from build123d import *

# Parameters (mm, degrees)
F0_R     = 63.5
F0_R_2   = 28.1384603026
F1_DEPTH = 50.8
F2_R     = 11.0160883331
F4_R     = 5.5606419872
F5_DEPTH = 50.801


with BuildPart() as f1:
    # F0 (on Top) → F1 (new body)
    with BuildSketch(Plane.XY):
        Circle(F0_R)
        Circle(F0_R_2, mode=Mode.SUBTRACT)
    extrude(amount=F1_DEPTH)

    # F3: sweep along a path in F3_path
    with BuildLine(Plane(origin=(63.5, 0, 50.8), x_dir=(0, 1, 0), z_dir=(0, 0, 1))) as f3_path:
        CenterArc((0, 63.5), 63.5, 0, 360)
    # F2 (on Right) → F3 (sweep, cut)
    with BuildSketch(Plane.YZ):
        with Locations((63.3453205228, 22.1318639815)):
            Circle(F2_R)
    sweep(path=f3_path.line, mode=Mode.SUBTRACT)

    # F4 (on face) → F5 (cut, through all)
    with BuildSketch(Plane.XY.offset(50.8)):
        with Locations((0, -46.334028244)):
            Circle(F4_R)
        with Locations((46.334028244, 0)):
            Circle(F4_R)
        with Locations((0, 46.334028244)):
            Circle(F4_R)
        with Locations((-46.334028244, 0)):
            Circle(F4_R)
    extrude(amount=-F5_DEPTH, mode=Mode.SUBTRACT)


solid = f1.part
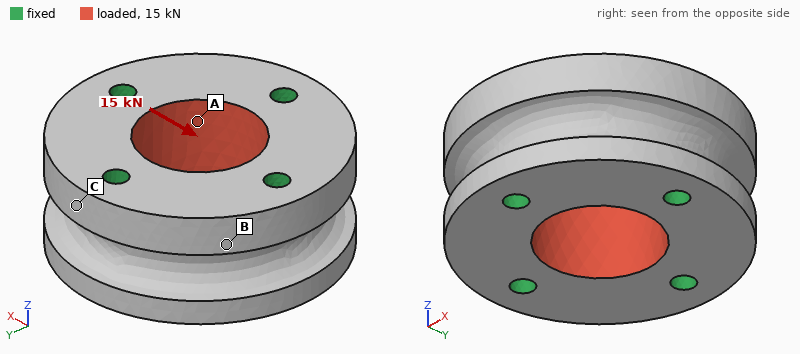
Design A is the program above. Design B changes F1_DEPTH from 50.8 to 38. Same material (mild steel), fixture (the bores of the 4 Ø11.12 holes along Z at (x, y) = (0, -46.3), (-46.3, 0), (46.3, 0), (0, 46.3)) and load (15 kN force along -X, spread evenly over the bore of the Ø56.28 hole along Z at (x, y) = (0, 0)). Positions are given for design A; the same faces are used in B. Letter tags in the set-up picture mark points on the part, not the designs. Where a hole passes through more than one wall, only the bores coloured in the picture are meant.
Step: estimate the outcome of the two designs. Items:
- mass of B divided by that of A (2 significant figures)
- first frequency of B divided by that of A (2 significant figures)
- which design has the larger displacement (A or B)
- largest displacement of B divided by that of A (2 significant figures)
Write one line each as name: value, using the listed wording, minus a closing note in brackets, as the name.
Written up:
mass of B divided by that of A: 0.71
first frequency of B divided by that of A: 0.95
which design has the larger displacement: B
largest displacement of B divided by that of A: 1.4
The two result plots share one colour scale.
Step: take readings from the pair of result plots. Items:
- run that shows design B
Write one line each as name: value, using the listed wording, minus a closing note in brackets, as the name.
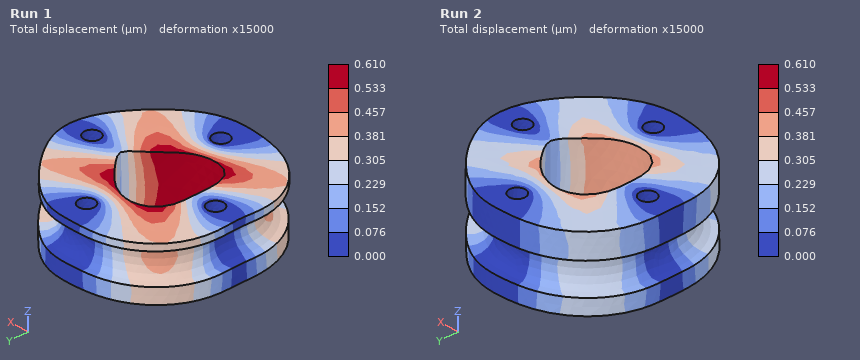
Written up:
run that shows design B: Run 1
